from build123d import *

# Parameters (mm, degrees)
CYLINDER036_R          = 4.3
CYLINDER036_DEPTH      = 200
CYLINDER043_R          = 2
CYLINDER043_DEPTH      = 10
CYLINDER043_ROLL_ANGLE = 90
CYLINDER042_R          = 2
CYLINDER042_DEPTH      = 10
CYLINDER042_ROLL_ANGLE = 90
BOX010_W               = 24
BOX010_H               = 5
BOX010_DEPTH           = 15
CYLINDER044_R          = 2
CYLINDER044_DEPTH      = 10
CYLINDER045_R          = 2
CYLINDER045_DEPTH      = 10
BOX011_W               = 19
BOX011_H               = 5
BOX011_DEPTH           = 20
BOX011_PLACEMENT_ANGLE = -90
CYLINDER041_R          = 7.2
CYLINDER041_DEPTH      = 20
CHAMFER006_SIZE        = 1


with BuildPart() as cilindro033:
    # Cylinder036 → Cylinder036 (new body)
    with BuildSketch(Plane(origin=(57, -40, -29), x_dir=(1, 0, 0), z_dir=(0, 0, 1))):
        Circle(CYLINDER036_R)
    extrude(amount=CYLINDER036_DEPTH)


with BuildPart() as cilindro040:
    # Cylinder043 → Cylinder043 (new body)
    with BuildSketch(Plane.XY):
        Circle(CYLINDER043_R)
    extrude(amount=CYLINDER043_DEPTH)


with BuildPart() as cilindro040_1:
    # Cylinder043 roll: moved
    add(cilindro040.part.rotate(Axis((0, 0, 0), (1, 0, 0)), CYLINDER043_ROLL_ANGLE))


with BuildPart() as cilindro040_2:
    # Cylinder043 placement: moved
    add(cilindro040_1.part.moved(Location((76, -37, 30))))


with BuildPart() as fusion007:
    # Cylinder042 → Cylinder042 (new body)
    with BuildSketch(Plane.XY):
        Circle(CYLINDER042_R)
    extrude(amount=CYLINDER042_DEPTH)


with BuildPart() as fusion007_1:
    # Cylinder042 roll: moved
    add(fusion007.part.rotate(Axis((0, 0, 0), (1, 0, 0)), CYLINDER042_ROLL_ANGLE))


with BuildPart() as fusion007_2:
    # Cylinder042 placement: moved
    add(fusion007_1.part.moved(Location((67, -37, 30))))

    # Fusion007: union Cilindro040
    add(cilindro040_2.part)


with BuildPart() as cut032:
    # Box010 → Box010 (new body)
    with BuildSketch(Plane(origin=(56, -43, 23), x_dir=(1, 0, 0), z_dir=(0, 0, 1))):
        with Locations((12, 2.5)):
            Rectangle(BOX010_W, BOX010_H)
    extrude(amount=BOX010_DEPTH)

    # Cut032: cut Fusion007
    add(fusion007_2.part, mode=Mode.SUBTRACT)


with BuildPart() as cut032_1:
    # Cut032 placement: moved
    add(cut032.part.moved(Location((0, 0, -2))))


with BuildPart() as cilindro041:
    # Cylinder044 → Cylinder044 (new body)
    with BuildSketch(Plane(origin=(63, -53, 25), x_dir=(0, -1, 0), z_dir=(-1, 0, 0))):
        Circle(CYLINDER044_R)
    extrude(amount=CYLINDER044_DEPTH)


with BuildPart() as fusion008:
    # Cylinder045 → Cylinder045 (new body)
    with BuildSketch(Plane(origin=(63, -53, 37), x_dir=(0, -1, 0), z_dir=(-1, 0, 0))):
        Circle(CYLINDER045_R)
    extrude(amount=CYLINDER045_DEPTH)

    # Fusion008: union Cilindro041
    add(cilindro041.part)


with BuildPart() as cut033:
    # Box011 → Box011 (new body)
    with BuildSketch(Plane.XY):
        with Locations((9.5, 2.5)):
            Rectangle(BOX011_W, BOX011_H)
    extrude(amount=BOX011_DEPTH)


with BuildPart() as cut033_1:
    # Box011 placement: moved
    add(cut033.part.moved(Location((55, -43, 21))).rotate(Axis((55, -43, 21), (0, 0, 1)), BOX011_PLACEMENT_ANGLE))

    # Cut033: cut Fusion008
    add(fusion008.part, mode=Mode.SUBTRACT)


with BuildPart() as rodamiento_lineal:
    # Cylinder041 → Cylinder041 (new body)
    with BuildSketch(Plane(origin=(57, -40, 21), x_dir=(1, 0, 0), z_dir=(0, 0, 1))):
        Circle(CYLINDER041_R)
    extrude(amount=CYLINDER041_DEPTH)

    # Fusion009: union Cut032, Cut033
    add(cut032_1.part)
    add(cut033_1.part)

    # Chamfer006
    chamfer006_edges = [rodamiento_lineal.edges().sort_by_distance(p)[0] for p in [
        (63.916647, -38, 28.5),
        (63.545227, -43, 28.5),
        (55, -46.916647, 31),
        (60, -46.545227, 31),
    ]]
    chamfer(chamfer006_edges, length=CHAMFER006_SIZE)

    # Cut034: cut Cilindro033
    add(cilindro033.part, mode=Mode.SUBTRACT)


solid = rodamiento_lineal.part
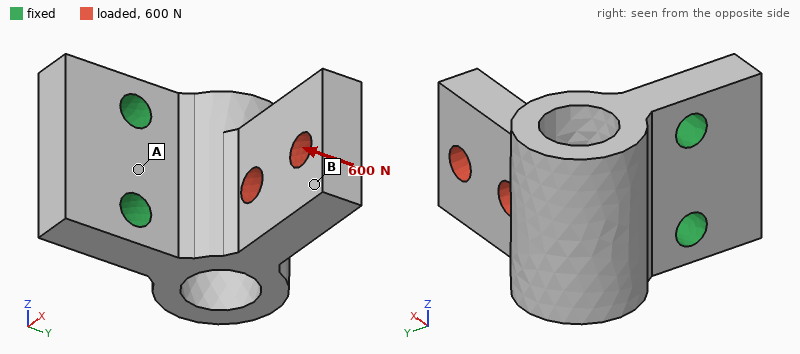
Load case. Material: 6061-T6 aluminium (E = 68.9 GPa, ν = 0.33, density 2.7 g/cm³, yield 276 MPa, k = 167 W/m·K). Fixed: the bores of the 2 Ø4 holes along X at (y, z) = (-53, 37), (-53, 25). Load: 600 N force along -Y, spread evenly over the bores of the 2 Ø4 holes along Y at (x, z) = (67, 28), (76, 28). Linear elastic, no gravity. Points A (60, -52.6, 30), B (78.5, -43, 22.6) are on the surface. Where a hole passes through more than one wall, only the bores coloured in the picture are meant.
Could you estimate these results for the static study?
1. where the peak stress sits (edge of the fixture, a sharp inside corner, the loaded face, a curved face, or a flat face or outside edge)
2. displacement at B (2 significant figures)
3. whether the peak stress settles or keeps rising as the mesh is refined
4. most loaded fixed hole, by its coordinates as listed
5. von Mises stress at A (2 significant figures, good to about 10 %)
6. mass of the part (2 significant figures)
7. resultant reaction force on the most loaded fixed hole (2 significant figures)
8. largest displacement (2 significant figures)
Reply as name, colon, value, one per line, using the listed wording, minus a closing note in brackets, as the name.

where the peak stress sits: edge of the fixture
displacement at B: 0.18 mm
whether the peak stress settles or keeps rising as the mesh is refined: keeps rising
most loaded fixed hole, by its coordinates as listed: (-53, 25)
von Mises stress at A: 41 MPa
mass of the part: 12 g
resultant reaction force on the most loaded fixed hole: 440 N
largest displacement: 0.21 mm
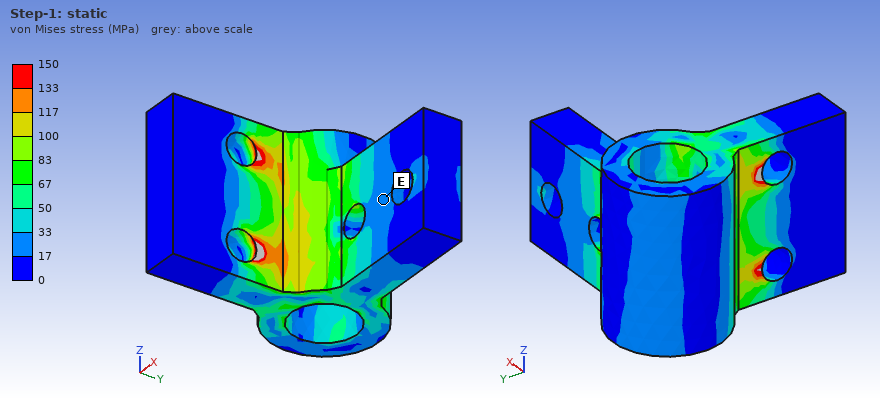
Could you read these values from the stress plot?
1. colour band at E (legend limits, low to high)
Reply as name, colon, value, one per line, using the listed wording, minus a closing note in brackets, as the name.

colour band at E: 17 to 33 MPa
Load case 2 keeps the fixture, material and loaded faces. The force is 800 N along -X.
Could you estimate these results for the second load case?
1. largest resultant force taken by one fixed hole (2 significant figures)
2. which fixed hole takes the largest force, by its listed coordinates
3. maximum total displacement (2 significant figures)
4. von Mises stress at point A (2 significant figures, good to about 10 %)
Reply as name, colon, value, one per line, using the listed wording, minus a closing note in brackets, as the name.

largest resultant force taken by one fixed hole: 560 N
which fixed hole takes the largest force, by its listed coordinates: (-53, 25)
maximum total displacement: 0.11 mm
von Mises stress at point A: 39 MPa
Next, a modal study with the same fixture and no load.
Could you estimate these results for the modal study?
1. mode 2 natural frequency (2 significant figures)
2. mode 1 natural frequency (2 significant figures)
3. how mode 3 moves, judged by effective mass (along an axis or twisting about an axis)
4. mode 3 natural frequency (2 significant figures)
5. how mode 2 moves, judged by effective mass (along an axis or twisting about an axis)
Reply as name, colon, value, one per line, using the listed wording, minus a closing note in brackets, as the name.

mode 2 natural frequency: 11 kHz
mode 1 natural frequency: 4800 Hz
how mode 3 moves, judged by effective mass: along X
mode 3 natural frequency: 15 kHz
how mode 2 moves, judged by effective mass: along Z
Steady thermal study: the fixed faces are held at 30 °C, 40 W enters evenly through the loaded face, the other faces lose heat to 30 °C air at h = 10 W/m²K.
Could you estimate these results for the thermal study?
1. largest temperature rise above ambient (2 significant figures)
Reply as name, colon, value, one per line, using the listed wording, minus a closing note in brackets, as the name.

largest temperature rise above ambient: 70 K
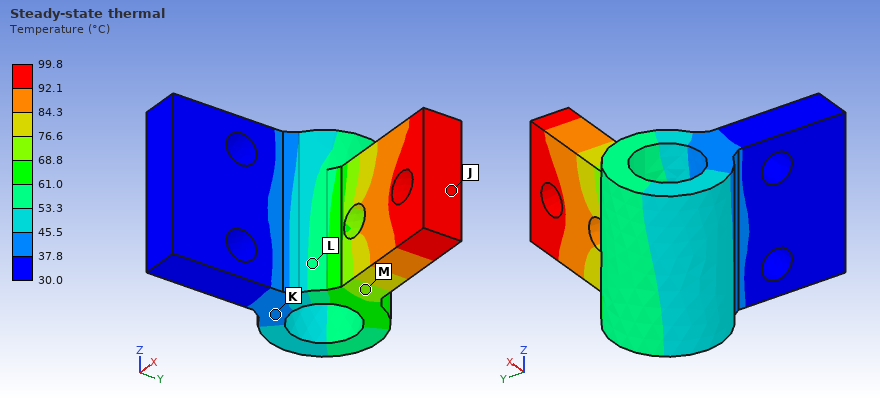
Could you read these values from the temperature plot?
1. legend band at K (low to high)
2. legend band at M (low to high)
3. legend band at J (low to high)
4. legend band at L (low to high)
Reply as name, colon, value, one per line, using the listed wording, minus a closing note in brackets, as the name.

legend band at K: 37.8 to 45.5 °C
legend band at M: 68.8 to 76.6 °C
legend band at J: 92.1 to 99.8 °C
legend band at L: 53.3 to 61.0 °C
